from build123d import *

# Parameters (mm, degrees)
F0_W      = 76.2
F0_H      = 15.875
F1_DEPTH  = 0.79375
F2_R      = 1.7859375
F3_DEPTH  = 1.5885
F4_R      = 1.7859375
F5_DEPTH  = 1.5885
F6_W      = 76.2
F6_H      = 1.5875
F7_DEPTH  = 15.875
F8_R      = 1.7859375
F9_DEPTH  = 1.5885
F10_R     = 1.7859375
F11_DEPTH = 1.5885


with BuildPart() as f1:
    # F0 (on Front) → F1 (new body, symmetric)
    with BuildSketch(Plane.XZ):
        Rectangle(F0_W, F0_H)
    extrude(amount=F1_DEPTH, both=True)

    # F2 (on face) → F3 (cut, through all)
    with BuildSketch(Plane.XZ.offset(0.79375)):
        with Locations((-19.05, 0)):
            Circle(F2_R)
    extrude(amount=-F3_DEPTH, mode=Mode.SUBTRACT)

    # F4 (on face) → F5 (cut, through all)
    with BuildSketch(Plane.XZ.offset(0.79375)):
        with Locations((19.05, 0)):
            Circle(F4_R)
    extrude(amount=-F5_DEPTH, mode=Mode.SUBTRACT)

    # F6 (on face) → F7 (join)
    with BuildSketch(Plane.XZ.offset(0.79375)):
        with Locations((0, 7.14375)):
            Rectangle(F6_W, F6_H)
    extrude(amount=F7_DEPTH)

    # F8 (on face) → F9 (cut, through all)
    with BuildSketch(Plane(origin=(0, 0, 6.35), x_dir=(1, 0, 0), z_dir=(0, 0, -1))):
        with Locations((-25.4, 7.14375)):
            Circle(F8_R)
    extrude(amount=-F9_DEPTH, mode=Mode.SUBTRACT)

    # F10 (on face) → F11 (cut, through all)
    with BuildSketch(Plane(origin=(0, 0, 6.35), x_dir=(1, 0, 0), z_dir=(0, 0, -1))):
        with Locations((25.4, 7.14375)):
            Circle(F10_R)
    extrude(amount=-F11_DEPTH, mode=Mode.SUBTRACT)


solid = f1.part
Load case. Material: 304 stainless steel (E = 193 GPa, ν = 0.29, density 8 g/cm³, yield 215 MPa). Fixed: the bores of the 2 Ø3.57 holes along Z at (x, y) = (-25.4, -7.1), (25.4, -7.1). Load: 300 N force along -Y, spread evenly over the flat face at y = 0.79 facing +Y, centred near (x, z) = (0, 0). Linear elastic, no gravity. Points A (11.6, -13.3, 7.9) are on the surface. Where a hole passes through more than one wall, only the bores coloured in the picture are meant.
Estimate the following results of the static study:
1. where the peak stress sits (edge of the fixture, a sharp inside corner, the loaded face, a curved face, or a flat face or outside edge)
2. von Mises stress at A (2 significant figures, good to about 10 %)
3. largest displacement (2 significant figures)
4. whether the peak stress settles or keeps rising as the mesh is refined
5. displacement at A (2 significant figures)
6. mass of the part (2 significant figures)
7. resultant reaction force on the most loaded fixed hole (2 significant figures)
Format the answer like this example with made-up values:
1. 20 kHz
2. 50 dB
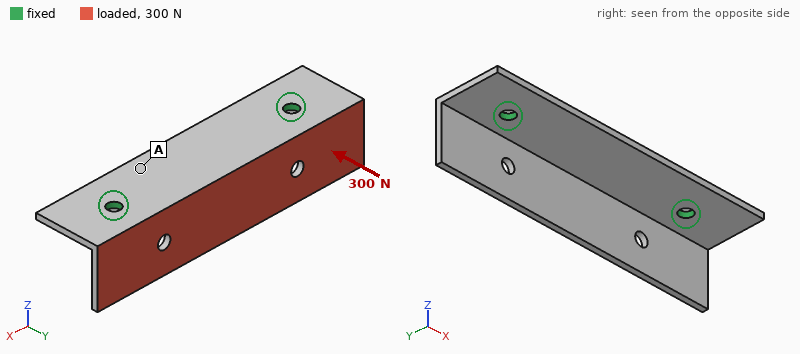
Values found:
1. edge of the fixture
2. 26 MPa
3. 94 µm
4. keeps rising
5. 22 µm
6. 30 g
7. 150 N
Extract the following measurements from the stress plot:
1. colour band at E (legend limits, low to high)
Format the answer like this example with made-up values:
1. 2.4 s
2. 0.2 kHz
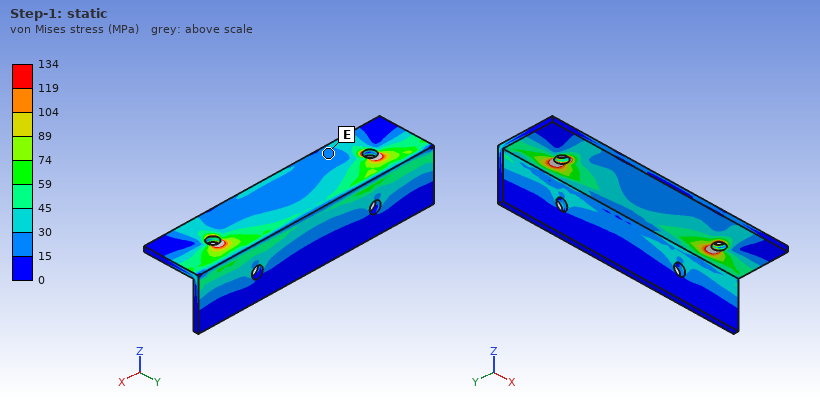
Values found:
1. 15 to 30 MPa
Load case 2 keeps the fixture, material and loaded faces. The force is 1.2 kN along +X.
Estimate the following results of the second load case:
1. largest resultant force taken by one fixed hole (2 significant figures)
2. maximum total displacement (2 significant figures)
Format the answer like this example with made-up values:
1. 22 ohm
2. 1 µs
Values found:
1. 640 N
2. 28 µm
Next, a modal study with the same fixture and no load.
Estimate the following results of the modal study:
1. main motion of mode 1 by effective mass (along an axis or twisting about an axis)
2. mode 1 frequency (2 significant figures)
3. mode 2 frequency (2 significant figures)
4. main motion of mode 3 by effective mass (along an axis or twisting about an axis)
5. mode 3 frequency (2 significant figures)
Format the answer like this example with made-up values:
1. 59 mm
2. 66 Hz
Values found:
1. along Y
2. 2700 Hz
3. 3800 Hz
4. along Z
5. 4600 Hz
